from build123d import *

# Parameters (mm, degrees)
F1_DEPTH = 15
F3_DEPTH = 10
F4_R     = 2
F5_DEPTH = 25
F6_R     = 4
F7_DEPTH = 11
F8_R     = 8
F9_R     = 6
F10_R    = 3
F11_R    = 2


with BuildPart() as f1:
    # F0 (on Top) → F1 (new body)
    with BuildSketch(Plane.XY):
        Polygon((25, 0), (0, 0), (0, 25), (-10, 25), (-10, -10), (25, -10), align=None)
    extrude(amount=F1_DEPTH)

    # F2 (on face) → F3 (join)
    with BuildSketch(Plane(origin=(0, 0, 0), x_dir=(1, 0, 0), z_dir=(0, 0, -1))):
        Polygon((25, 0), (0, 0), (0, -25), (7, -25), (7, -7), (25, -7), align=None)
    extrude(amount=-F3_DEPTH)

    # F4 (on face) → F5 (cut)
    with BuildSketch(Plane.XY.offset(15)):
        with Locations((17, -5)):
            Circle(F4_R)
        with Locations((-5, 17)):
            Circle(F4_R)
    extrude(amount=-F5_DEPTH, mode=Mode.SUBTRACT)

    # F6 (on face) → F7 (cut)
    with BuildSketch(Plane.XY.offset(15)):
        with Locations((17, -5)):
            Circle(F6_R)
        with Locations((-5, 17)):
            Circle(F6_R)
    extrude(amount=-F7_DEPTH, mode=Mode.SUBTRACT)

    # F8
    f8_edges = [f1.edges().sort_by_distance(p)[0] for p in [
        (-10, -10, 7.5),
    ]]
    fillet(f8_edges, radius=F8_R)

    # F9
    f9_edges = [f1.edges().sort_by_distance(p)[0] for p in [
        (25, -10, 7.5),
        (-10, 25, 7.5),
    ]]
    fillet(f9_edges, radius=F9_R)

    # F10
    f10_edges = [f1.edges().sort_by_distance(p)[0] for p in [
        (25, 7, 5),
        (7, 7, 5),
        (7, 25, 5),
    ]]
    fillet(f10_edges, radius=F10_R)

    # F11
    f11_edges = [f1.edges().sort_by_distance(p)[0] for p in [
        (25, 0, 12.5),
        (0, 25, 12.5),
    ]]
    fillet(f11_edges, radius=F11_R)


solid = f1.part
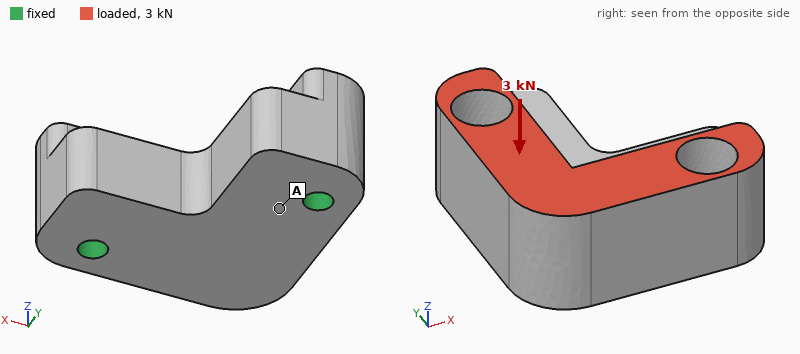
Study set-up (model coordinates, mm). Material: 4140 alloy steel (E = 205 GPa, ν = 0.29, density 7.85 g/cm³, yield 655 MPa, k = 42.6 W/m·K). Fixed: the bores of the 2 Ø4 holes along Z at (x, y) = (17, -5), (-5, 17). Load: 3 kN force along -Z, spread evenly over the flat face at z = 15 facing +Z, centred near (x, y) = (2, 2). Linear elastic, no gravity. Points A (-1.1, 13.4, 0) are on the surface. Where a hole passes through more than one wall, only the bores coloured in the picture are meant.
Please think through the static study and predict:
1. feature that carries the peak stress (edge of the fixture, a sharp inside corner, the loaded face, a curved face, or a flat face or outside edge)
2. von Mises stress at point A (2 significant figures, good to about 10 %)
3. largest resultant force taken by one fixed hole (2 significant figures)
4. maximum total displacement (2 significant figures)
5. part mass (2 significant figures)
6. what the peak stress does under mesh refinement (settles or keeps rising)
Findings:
edge of the fixture
34 MPa
1.6 kN
25 µm
81 g
keeps rising
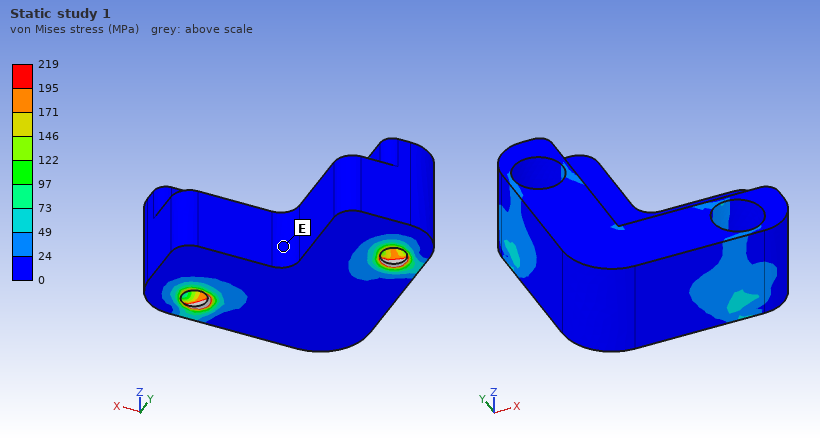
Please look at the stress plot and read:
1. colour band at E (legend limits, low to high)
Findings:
0 to 24 MPa
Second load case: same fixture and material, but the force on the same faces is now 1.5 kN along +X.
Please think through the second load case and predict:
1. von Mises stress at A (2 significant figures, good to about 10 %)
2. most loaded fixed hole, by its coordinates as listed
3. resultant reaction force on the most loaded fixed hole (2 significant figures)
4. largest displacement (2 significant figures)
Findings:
18 MPa
(17, -5)
1.1 kN
17 µm
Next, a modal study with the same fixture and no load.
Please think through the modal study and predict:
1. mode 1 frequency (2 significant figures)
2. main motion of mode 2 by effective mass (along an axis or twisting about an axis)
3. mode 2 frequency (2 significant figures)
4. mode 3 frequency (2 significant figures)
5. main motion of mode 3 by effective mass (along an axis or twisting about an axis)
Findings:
7700 Hz
along Z
21 kHz
24 kHz
twisting about Z
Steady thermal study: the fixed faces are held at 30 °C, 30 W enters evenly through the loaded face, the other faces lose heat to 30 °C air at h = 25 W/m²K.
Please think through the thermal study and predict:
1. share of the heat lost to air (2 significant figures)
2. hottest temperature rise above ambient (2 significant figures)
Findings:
7.1 %
44 K
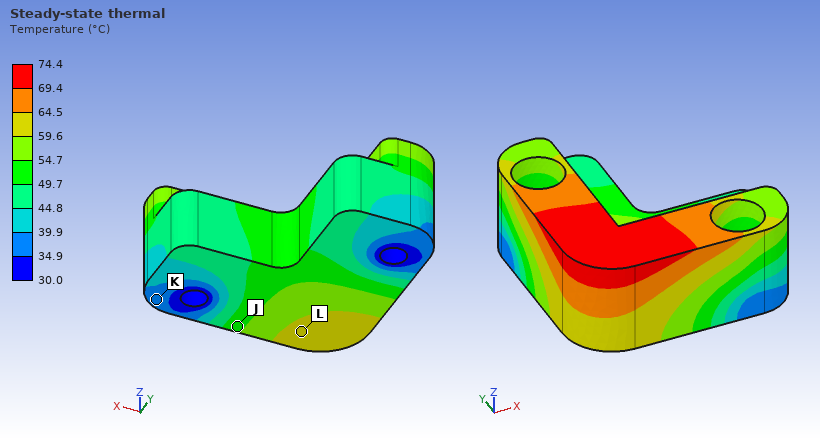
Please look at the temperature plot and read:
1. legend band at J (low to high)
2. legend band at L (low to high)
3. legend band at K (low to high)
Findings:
49.7 to 54.7 °C
59.6 to 64.5 °C
34.9 to 39.9 °C
